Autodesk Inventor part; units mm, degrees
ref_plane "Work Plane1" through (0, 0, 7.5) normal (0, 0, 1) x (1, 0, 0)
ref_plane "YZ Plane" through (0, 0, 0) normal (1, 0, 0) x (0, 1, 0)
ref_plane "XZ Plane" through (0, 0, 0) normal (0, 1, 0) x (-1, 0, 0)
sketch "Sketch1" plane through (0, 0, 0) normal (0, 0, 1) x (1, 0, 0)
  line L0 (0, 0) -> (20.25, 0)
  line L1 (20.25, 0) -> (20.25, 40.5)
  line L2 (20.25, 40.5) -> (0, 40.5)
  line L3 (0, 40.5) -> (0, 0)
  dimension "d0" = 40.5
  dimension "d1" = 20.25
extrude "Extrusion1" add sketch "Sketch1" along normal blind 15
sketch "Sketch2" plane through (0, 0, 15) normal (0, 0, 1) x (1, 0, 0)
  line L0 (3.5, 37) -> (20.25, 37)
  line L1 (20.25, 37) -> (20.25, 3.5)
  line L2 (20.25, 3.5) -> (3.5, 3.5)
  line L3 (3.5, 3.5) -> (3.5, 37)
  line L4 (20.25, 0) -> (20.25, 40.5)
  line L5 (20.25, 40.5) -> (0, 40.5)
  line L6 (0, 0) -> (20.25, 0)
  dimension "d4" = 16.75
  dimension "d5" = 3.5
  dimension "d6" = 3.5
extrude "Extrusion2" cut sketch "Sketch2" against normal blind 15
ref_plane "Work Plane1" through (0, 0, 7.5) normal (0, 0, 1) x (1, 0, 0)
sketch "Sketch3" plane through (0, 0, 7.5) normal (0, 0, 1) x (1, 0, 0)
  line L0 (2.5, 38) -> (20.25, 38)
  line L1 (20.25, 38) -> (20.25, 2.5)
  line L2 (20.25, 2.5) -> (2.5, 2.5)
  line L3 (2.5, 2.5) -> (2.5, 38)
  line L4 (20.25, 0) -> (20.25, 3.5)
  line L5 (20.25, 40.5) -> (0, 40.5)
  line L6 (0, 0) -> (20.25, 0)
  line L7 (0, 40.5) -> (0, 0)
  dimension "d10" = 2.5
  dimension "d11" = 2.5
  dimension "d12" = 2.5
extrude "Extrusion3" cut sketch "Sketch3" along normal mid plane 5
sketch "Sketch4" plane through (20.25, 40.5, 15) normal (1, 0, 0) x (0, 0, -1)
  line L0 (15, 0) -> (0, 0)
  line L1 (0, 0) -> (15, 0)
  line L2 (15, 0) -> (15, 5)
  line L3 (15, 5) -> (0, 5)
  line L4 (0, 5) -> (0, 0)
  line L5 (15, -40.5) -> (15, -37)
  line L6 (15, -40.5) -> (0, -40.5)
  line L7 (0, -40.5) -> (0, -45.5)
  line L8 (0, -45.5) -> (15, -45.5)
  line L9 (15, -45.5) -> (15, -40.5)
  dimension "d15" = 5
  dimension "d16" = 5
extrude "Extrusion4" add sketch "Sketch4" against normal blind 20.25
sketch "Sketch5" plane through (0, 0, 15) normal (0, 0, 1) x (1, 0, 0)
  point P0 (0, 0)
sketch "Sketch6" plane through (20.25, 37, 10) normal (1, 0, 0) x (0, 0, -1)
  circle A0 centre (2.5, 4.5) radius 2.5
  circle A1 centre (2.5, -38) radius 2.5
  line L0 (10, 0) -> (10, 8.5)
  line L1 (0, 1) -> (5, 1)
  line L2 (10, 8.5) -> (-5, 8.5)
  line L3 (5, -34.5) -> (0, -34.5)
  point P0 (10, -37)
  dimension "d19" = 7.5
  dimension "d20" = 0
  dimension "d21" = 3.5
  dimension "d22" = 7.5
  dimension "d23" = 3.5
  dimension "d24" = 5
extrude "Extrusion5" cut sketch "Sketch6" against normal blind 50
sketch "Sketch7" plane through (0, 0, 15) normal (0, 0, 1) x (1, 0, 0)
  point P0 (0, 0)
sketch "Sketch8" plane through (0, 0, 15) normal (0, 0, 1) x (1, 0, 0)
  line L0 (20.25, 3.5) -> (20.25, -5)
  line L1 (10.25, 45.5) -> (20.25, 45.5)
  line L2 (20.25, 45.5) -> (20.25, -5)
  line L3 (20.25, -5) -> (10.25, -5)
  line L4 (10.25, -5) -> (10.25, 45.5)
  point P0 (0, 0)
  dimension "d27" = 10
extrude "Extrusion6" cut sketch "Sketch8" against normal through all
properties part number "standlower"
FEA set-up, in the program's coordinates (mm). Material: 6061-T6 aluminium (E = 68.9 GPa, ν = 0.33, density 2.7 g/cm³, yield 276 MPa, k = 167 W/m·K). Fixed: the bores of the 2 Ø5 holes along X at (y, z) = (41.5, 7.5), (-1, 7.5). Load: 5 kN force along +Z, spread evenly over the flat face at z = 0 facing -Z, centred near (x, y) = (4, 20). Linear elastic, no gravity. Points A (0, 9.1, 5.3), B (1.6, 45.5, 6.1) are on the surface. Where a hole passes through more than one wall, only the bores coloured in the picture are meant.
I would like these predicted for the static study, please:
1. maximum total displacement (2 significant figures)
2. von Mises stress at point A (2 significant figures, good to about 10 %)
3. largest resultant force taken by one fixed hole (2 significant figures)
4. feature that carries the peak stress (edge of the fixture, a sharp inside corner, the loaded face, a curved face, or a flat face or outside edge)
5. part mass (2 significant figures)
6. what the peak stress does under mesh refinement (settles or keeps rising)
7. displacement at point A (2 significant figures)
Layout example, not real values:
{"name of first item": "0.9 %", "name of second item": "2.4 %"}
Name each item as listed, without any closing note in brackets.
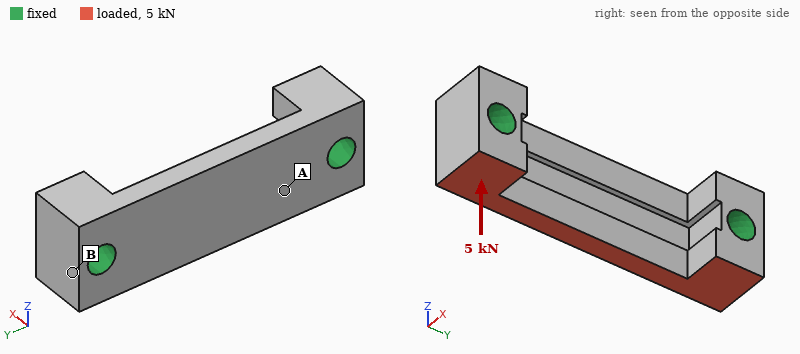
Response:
{"maximum total displacement": "28 µm", "von Mises stress at point A": "27 MPa", "largest resultant force taken by one fixed hole": "2.5 kN", "feature that carries the peak stress": "edge of the fixture", "part mass": "10 g", "what the peak stress does under mesh refinement": "keeps rising", "displacement at point A": "13 µm"}
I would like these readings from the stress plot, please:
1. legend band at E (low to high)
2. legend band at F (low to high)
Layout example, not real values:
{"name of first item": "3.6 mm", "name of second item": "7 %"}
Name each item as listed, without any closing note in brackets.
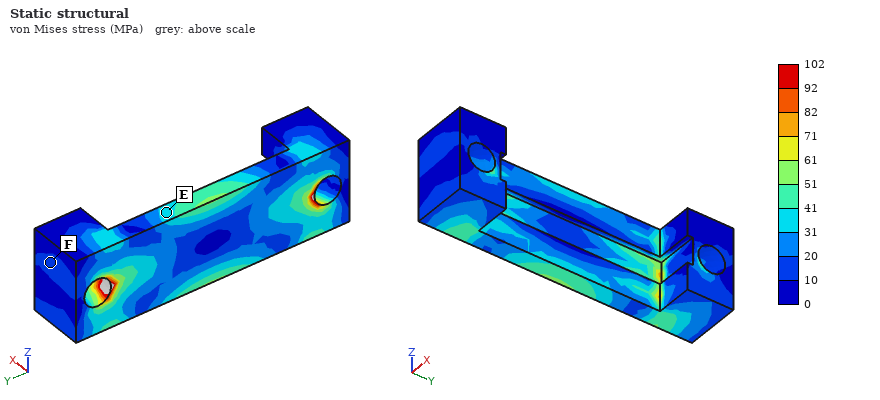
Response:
{"legend band at E": "31 to 41 MPa", "legend band at F": "10 to 20 MPa"}
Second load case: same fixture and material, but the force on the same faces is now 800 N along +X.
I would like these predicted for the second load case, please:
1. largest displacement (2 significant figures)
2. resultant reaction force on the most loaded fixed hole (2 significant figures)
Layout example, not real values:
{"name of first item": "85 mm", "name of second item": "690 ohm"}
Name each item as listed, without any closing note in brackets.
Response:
{"largest displacement": "37 µm", "resultant reaction force on the most loaded fixed hole": "400 N"}
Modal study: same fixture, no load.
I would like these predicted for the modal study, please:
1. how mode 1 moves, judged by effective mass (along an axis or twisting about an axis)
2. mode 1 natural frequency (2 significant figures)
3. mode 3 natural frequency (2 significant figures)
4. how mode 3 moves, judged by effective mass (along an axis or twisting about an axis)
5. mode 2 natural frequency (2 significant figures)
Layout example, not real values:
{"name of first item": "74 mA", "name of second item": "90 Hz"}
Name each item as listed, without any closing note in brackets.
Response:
{"how mode 1 moves, judged by effective mass": "along X", "mode 1 natural frequency": "12 kHz", "mode 3 natural frequency": "26 kHz", "how mode 3 moves, judged by effective mass": "along Z", "mode 2 natural frequency": "19 kHz"}
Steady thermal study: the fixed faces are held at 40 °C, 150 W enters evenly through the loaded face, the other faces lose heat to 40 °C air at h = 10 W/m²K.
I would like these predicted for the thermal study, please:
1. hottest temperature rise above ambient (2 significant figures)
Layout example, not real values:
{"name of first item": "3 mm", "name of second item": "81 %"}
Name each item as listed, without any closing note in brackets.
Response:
{"hottest temperature rise above ambient": "63 K"}
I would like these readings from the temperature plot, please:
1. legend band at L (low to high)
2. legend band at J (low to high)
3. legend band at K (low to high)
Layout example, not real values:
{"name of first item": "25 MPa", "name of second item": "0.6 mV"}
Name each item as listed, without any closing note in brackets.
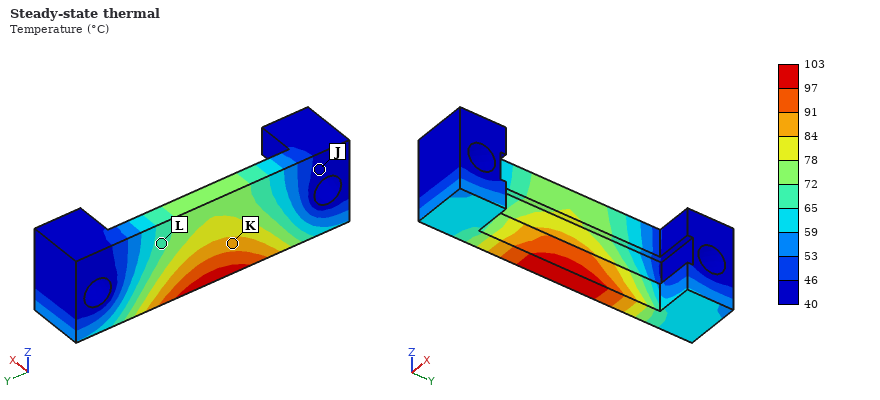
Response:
{"legend band at L": "65 to 72 °C", "legend band at J": "40 to 46 °C", "legend band at K": "84 to 91 °C"}
